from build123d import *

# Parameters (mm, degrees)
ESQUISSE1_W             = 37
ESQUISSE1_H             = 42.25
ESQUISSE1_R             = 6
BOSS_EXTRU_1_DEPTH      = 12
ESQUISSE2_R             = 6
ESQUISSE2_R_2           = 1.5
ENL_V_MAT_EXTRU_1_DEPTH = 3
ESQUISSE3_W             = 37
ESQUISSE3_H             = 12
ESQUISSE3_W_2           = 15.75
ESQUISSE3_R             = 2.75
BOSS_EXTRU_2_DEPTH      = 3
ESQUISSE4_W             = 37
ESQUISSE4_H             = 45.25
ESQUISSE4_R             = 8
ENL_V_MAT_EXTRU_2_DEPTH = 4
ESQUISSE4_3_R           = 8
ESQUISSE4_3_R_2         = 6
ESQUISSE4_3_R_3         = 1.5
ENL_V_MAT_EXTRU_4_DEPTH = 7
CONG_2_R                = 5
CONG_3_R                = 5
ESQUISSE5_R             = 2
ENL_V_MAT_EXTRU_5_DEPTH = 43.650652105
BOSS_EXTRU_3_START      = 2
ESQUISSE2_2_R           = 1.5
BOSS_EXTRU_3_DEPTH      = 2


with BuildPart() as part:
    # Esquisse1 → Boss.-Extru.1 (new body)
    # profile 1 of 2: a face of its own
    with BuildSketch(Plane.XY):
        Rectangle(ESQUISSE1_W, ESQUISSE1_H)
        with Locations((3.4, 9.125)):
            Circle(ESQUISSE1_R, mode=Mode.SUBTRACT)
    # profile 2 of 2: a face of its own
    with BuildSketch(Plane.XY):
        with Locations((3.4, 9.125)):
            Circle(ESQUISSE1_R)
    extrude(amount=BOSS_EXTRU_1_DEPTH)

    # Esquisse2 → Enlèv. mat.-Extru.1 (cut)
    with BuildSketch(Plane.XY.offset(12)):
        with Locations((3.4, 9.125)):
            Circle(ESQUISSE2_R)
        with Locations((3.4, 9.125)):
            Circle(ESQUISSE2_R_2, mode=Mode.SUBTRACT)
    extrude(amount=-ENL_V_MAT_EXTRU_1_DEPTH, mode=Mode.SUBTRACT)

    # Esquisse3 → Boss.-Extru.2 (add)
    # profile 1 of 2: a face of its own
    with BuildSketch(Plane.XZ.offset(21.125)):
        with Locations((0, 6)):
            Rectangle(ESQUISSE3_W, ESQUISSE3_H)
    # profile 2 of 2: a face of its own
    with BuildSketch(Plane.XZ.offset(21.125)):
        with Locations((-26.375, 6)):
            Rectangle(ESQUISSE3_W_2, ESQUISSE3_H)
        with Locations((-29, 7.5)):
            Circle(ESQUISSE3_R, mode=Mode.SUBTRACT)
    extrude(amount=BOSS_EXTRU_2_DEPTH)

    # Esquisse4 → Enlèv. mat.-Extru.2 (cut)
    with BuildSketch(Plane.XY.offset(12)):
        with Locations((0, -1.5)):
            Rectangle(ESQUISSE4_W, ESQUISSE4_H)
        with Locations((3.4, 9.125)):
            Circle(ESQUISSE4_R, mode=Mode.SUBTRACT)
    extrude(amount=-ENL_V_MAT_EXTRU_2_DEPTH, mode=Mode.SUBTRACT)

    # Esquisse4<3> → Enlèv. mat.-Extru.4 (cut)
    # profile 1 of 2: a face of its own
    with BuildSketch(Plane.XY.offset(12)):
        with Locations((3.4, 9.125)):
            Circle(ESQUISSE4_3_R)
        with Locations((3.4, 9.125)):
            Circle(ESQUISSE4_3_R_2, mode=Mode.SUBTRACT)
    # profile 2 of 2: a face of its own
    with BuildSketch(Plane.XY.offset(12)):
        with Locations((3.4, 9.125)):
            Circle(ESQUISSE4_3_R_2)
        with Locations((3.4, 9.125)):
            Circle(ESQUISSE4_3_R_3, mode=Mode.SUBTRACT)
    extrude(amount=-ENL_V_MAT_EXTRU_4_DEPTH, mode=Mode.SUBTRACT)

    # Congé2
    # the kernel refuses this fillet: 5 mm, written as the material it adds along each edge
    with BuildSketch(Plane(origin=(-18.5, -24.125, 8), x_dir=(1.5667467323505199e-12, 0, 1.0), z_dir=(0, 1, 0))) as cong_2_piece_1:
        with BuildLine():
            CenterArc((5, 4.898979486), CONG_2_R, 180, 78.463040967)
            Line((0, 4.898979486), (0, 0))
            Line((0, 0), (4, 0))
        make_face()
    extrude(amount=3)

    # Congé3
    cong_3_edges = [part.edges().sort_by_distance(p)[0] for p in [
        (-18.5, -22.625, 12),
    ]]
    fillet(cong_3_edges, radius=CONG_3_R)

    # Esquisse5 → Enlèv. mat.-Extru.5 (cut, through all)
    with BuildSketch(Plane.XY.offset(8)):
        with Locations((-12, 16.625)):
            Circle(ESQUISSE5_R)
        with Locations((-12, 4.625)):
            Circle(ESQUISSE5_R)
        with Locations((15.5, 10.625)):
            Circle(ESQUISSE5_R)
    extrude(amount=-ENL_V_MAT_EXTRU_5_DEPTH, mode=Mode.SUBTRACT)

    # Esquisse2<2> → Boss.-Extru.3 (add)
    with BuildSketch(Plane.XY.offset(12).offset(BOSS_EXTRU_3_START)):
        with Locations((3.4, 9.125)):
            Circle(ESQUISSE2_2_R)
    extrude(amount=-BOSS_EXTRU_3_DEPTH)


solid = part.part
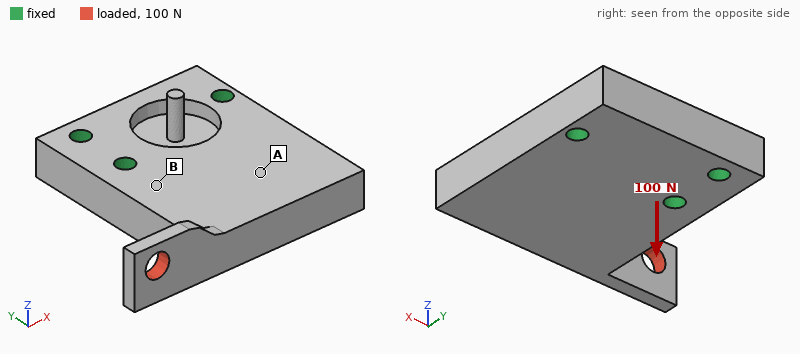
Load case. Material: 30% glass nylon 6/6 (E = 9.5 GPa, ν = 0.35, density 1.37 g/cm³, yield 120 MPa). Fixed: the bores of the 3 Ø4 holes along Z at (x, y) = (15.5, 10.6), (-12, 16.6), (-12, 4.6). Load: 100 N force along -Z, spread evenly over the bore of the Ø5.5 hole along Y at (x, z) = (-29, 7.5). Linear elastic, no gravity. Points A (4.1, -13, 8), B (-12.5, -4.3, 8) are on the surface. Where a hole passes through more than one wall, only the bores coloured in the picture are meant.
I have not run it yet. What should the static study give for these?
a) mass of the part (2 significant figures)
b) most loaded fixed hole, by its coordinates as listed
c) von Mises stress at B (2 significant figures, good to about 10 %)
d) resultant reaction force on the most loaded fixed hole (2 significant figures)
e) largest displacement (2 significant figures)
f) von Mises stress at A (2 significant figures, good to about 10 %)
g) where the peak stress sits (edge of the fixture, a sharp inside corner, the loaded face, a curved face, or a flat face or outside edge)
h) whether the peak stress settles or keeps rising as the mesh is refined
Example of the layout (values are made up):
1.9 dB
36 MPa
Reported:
18 g
(-12, 4.6)
10 MPa
190 N
0.31 mm
4.6 MPa
edge of the fixture
keeps rising
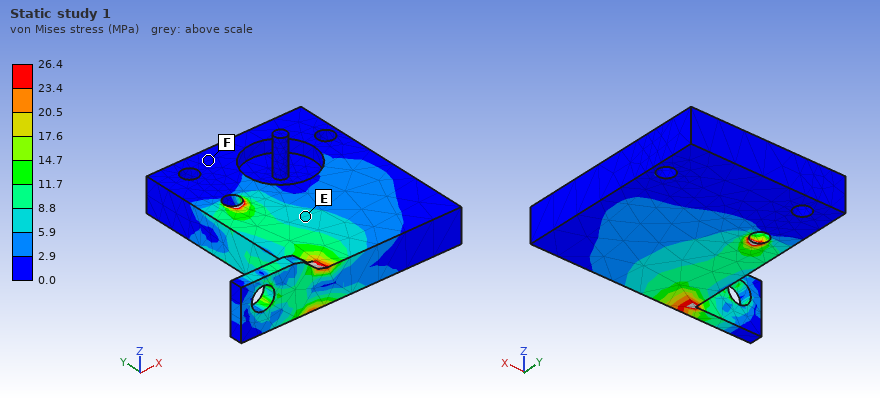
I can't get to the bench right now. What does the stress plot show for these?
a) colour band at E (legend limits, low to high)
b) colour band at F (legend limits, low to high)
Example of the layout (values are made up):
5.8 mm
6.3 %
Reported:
5.9 to 8.8 MPa
0.0 to 2.9 MPa
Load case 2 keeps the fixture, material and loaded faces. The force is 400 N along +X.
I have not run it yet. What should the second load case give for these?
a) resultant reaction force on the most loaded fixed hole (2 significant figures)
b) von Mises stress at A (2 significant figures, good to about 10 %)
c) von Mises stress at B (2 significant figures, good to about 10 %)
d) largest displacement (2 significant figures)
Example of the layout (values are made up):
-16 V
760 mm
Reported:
450 N
5.6 MPa
5.8 MPa
0.23 mm
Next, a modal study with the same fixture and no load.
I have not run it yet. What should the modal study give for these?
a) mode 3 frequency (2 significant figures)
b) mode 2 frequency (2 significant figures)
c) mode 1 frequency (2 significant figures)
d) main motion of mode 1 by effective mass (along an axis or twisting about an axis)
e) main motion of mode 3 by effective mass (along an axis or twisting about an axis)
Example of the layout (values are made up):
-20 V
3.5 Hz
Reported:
4200 Hz
4000 Hz
2800 Hz
along Z
twisting about Y
